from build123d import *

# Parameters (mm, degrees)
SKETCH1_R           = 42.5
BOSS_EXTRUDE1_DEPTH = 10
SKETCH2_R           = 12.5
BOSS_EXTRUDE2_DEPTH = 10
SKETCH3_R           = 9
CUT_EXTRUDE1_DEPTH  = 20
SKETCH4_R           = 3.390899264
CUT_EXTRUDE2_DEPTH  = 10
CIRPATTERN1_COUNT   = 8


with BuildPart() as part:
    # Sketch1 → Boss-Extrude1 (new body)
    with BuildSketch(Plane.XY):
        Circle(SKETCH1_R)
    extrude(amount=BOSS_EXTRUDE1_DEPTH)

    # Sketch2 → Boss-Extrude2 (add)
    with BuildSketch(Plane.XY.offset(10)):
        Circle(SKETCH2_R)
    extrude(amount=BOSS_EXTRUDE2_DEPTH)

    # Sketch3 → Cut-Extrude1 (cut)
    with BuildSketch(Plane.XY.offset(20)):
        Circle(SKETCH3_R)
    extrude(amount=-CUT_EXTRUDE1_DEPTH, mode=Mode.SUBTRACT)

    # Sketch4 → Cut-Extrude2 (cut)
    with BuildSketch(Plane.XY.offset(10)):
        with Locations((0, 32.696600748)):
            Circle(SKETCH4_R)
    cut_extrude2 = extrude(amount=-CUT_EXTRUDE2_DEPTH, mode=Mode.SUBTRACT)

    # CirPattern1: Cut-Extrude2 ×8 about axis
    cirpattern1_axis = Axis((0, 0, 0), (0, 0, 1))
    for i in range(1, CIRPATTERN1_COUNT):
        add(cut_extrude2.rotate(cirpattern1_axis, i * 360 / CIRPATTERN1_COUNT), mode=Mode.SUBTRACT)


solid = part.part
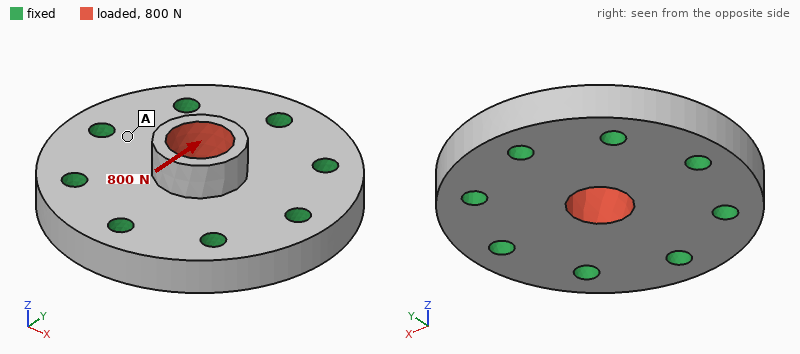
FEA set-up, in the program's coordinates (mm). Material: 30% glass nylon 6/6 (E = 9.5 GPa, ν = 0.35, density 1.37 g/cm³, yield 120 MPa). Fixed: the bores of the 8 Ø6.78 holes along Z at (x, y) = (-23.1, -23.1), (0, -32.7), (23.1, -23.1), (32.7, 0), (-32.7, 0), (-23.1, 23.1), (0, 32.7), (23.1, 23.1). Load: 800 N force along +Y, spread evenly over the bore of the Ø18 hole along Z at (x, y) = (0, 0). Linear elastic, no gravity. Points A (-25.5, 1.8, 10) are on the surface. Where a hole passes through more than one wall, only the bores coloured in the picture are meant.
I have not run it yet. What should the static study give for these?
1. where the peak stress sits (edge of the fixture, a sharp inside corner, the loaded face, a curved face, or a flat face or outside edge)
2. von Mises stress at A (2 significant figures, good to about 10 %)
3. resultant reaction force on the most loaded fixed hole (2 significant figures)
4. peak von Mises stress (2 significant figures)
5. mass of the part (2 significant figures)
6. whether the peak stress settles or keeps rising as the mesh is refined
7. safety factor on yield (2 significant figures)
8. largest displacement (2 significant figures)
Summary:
the loaded face
0.47 MPa
180 N
4.7 MPa
74 g
settles
26
13 µm
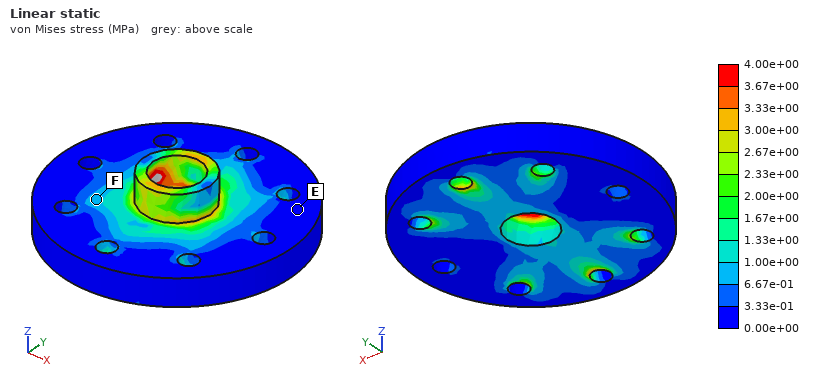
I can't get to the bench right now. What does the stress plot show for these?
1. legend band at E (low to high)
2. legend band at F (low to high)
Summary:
0.00e+00 to 3.33e-01 MPa
6.67e-01 to 1.00e+00 MPa
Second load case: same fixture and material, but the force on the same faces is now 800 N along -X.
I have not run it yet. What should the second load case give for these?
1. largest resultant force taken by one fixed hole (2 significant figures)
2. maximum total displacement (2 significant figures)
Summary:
180 N
13 µm
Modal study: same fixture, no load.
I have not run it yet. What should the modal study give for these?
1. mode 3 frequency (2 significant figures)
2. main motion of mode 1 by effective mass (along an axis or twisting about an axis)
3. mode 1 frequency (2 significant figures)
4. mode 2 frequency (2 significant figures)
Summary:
14 kHz
along Z
10 kHz
14 kHz
